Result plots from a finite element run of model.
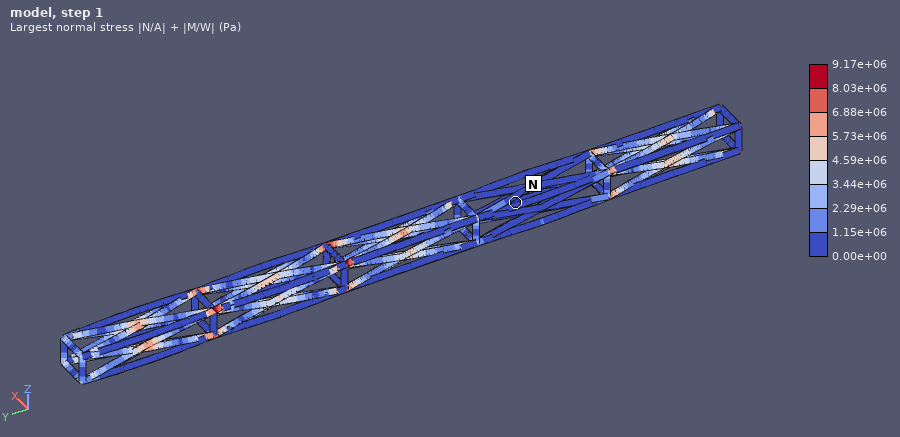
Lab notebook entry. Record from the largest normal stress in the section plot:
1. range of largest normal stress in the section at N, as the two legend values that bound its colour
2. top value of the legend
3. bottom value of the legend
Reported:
0.00e+00 to 1.15e+06 Pa
9.17e+06 Pa
0.00e+00 Pa
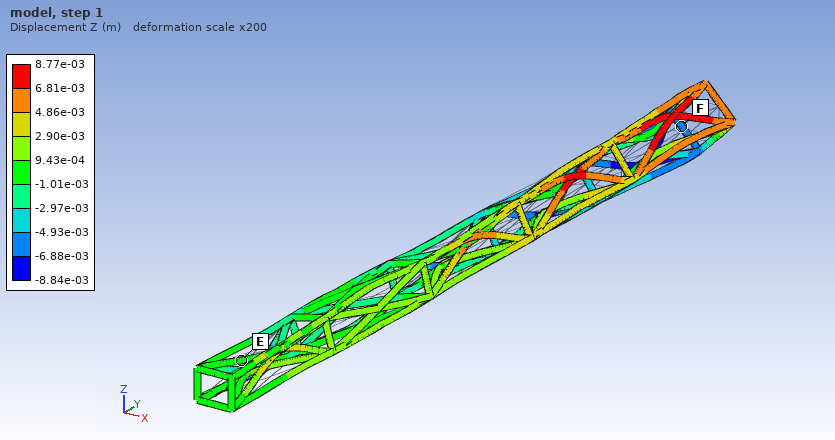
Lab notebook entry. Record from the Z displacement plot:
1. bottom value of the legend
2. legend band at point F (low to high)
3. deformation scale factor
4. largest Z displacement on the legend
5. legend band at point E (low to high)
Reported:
-8.84e-03 m
-6.88e-03 to -4.93e-03 m
200
8.77e-03 m
-1.01e-03 to 9.43e-04 m
